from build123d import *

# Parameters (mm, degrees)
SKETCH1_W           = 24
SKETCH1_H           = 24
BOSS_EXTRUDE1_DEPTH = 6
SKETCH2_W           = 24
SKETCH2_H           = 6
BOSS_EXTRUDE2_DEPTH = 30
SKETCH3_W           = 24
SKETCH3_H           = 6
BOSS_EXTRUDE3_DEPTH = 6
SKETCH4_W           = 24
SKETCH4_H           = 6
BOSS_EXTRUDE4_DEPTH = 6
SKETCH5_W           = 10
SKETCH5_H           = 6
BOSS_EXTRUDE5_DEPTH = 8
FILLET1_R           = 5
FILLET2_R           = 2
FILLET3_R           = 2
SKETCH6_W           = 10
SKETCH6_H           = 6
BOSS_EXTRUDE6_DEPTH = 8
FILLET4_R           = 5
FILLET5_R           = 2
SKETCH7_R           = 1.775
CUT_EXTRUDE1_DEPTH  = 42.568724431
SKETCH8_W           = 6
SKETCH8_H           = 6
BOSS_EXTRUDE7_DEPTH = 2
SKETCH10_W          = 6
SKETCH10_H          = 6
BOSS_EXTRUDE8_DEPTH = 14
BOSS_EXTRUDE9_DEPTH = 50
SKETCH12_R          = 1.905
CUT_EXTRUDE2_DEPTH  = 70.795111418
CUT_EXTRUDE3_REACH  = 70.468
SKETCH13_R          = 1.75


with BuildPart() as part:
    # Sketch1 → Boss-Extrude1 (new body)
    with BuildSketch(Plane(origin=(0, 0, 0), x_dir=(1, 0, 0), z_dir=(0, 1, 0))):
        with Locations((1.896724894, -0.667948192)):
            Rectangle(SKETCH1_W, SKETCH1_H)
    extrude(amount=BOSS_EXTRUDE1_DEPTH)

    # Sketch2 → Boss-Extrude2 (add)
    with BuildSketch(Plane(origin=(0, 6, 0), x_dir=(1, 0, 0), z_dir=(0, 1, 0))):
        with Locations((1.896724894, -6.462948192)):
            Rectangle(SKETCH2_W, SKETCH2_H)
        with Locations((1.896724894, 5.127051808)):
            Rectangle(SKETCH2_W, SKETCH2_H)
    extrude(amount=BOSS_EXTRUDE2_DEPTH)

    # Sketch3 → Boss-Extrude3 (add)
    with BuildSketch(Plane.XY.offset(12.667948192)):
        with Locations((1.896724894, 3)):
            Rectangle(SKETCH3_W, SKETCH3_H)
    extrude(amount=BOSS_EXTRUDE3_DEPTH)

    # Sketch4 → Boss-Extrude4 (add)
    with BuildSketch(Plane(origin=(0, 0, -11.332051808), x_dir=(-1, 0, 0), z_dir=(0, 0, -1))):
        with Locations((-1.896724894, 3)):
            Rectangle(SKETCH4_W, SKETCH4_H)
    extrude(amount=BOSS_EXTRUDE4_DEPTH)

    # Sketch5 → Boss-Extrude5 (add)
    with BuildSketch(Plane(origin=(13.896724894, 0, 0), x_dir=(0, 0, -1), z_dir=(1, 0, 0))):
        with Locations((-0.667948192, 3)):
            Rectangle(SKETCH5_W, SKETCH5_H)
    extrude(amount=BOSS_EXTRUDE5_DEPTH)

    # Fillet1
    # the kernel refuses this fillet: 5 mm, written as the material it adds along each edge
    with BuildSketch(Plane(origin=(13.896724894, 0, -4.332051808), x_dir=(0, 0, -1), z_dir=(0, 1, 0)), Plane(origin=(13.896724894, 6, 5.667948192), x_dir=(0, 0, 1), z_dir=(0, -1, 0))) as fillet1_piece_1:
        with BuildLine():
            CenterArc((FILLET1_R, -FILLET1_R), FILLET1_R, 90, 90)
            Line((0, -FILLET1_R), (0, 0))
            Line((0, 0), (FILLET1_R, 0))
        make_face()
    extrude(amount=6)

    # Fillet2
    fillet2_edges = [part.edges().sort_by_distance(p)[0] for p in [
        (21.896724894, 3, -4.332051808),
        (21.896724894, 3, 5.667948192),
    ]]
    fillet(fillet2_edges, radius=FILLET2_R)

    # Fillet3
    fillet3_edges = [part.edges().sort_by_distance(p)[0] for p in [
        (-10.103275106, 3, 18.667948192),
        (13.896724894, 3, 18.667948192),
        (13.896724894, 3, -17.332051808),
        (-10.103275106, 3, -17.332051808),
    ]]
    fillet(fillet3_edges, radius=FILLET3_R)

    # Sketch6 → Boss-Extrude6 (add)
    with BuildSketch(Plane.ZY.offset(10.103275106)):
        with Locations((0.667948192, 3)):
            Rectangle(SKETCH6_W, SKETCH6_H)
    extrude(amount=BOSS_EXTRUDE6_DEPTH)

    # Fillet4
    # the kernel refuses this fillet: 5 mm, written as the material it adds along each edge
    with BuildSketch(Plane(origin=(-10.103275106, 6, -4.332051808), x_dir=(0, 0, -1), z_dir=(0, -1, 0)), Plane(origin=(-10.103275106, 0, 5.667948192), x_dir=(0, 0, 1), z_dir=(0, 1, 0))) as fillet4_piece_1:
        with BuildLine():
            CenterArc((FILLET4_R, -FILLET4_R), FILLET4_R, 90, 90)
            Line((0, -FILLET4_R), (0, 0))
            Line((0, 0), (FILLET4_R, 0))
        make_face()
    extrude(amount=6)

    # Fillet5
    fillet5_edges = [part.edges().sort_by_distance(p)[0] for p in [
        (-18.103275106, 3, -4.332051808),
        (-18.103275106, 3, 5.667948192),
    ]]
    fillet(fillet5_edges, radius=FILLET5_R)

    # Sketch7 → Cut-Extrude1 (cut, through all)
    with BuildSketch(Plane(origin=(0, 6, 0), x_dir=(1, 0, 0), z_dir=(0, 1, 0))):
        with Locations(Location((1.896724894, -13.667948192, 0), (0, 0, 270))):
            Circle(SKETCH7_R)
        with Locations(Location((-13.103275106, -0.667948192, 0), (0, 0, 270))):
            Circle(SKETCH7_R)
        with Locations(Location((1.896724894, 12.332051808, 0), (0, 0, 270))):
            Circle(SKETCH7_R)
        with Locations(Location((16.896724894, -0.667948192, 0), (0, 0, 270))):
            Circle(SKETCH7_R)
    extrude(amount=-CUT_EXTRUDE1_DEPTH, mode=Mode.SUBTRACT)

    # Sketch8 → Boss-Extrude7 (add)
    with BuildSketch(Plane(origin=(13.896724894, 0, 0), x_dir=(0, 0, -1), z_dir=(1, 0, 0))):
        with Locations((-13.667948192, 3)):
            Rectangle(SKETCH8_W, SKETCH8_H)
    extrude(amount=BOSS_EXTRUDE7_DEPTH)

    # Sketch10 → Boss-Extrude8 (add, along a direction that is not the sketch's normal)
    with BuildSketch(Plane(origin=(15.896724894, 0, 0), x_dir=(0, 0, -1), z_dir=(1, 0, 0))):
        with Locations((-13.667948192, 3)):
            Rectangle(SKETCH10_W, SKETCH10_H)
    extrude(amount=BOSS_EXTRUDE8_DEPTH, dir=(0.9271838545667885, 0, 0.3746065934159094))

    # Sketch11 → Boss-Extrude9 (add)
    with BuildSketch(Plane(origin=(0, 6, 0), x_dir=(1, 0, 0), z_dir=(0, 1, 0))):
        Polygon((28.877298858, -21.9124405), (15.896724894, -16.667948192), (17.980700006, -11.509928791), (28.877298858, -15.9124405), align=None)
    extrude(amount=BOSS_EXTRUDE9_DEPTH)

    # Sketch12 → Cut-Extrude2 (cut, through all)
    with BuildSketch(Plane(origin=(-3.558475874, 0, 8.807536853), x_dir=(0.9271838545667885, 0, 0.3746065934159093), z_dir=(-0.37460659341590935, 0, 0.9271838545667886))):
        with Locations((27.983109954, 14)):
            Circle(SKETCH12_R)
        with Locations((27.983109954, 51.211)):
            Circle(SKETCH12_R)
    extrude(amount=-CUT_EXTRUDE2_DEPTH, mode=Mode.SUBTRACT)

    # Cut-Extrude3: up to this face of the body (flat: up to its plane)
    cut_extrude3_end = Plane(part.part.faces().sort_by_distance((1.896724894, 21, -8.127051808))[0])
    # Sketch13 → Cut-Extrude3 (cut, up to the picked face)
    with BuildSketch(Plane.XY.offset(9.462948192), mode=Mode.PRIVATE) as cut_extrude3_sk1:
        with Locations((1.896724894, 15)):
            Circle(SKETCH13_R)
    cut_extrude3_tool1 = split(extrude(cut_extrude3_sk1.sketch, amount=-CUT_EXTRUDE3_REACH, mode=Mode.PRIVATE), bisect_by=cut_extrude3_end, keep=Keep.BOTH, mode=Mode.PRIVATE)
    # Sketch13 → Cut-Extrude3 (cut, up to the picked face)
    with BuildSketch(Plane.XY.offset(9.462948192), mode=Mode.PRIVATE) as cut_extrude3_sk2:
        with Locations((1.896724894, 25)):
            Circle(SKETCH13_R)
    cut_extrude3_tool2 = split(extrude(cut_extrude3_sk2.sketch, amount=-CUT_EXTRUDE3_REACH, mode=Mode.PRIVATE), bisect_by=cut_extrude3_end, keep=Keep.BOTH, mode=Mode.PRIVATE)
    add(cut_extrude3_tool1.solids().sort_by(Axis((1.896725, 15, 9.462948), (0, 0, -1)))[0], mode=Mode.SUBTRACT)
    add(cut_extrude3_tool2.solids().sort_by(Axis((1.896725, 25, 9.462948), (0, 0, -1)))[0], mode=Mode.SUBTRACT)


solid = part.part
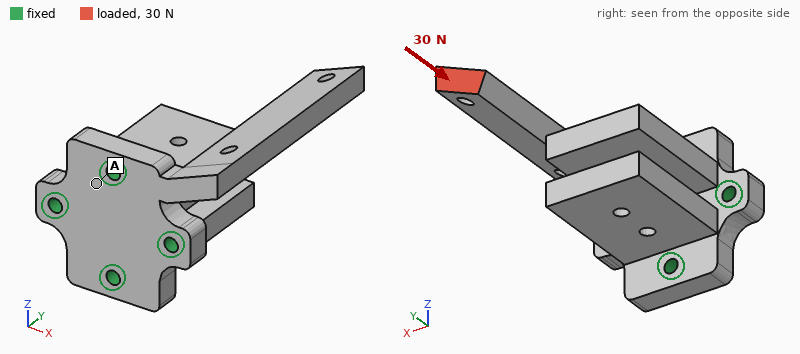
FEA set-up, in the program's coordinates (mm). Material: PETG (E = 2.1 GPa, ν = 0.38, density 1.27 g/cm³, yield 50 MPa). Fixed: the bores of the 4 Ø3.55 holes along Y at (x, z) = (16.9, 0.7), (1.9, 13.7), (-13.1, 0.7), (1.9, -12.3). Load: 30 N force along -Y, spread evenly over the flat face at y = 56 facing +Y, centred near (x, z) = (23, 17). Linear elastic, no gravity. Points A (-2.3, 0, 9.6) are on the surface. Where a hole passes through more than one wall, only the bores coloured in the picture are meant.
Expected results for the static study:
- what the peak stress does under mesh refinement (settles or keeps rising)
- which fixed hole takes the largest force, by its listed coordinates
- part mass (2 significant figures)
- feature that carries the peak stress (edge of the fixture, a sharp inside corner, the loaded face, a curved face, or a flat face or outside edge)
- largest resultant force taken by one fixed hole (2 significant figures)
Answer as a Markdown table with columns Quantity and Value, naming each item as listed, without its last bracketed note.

| Quantity | Value |
|---|---|
| what the peak stress does under mesh refinement | keeps rising |
| which fixed hole takes the largest force, by its listed coordinates | (1.9, 13.7) |
| part mass | 23 g |
| feature that carries the peak stress | a sharp inside corner |
| largest resultant force taken by one fixed hole | 26 N |
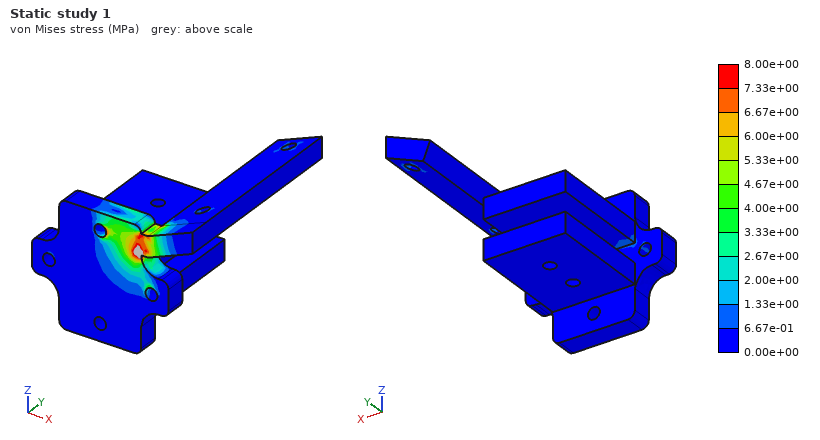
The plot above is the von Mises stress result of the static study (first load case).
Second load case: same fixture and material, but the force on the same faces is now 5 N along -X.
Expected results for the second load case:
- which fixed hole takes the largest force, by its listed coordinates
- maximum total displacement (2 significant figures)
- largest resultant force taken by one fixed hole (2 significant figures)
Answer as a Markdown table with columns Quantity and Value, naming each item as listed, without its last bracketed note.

| Quantity | Value |
|---|---|
| which fixed hole takes the largest force, by its listed coordinates | (16.9, 0.7) |
| maximum total displacement | 0.95 mm |
| largest resultant force taken by one fixed hole | 9.9 N |
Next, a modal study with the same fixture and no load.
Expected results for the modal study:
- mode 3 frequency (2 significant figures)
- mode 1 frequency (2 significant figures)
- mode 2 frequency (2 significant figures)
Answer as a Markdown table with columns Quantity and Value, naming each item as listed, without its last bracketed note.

| Quantity | Value |
|---|---|
| mode 3 frequency | 1100 Hz |
| mode 1 frequency | 250 Hz |
| mode 2 frequency | 310 Hz |
